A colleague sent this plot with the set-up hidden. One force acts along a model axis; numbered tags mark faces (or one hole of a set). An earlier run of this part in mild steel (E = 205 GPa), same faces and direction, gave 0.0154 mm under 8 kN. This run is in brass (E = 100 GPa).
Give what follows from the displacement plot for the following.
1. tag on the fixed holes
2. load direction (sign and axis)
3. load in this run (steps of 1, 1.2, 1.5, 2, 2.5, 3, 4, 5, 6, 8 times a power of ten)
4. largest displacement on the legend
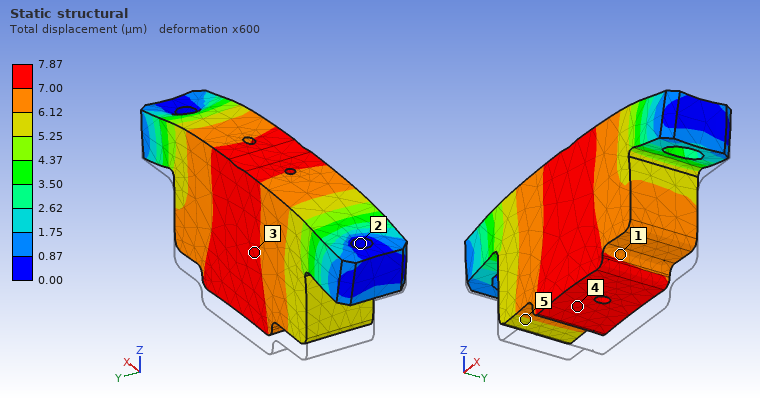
2
+Z
2 kN
7.87 µm
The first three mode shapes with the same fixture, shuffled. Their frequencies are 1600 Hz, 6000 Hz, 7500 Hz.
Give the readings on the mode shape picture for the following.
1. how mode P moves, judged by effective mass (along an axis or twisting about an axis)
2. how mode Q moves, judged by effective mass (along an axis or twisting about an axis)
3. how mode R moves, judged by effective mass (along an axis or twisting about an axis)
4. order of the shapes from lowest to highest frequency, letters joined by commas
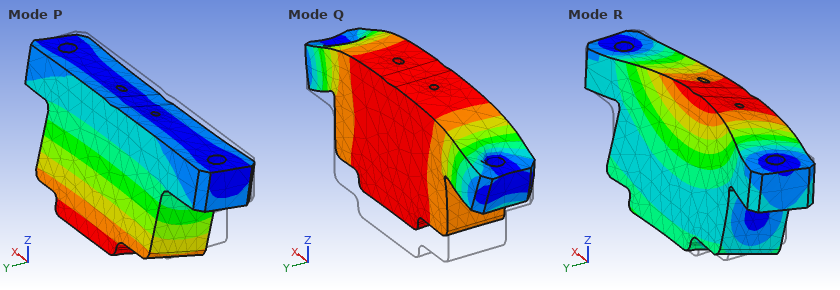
along Y
along Z
along Y
P, Q, R
